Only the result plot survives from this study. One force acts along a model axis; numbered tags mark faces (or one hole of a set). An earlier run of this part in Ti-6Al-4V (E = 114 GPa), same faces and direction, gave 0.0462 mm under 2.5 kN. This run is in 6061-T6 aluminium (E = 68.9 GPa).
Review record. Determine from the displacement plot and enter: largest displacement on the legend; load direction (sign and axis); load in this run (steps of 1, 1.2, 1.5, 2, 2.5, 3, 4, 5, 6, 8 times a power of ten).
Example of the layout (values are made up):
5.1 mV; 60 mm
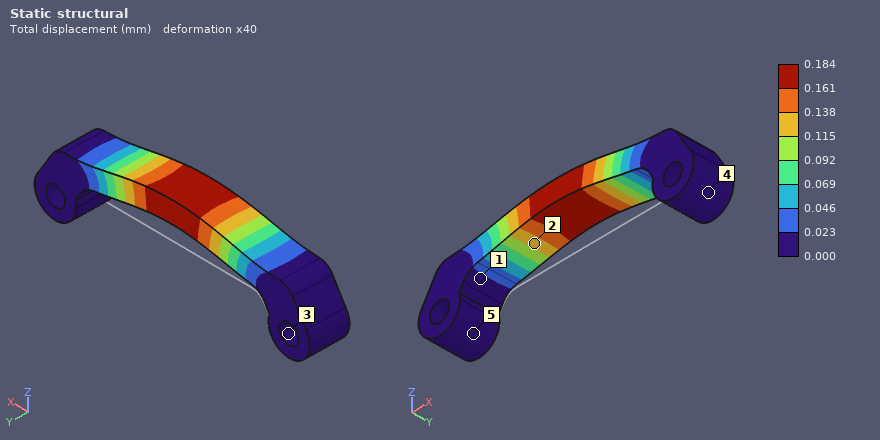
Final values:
0.184 mm; +Z; 6 kN
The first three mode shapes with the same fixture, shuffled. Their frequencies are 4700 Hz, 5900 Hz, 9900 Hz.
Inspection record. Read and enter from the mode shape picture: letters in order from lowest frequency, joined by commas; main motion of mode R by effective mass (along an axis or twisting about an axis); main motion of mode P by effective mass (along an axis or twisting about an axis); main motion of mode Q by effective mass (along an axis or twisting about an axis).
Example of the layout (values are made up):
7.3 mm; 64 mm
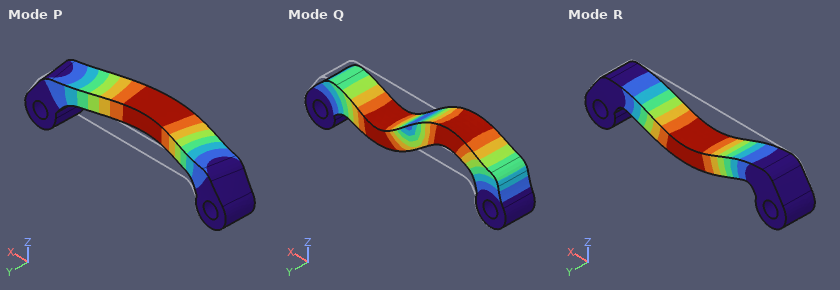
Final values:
R, P, Q; along Z; along Y; along X
